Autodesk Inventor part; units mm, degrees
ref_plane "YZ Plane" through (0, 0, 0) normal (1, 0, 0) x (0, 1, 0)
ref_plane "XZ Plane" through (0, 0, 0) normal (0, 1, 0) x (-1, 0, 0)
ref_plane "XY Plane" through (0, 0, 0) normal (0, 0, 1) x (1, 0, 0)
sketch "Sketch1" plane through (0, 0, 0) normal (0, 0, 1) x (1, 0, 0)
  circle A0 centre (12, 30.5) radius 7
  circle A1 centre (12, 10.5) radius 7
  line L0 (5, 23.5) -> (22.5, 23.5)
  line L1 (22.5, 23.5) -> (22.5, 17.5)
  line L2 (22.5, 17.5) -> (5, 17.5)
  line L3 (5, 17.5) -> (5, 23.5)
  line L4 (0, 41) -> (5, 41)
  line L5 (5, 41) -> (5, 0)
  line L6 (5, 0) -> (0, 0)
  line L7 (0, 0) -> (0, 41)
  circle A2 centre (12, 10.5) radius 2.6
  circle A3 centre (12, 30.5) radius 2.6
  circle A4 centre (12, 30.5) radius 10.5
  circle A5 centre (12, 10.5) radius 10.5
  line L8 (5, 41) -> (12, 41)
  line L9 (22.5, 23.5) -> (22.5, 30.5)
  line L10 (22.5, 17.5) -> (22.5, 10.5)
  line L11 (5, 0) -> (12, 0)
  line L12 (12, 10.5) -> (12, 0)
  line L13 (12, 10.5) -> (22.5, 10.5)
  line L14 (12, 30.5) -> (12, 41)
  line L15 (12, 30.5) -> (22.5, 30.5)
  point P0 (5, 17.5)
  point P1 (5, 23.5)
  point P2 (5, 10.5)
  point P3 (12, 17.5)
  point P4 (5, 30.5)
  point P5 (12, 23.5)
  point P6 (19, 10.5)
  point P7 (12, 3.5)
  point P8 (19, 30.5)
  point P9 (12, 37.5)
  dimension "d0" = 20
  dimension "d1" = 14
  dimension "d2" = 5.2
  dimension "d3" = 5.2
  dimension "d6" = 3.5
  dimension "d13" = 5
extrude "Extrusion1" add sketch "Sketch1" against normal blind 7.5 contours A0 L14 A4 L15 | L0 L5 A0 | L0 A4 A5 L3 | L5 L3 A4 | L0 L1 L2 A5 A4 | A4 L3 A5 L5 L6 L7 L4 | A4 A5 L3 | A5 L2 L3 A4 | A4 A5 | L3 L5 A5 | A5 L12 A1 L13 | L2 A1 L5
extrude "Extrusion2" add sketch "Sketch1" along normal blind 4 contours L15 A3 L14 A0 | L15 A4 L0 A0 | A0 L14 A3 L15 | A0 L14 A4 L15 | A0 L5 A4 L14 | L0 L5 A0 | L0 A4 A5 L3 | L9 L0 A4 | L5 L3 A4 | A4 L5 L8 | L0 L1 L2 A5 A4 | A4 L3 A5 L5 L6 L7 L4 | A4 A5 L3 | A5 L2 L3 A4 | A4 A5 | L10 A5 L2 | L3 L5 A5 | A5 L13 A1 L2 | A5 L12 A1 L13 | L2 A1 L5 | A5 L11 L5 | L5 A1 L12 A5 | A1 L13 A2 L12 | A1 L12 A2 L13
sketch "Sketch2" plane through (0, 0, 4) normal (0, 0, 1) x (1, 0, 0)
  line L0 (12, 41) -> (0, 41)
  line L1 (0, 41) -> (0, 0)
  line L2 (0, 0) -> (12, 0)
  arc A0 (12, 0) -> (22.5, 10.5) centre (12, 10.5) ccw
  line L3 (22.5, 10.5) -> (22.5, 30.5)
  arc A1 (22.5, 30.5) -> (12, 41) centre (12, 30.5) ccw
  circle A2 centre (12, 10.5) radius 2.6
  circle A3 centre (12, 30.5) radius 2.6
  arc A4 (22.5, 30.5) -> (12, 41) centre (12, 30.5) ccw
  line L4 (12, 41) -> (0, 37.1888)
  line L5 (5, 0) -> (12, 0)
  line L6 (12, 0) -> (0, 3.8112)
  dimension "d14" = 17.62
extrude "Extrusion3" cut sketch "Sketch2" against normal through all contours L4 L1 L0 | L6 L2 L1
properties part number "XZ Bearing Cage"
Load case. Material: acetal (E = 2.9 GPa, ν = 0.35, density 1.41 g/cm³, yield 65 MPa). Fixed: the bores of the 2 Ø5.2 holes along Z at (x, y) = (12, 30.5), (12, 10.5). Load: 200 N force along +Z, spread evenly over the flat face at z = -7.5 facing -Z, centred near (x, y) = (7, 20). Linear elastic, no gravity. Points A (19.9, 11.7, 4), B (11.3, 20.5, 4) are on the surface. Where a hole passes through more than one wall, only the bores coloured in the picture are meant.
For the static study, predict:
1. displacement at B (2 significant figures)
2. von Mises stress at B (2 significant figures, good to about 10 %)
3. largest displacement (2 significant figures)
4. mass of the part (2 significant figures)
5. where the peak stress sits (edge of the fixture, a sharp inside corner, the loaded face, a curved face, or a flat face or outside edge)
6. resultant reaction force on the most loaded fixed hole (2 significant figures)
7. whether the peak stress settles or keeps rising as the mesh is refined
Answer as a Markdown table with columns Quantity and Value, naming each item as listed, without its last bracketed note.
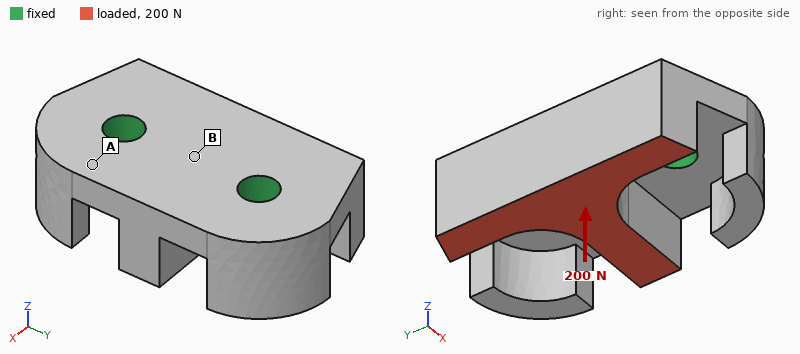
| Quantity | Value |
|---|---|
| displacement at B | 13 µm |
| von Mises stress at B | 2.4 MPa |
| largest displacement | 64 µm |
| mass of the part | 8.6 g |
| where the peak stress sits | edge of the fixture |
| resultant reaction force on the most loaded fixed hole | 100 N |
| whether the peak stress settles or keeps rising as the mesh is refined | keeps rising |
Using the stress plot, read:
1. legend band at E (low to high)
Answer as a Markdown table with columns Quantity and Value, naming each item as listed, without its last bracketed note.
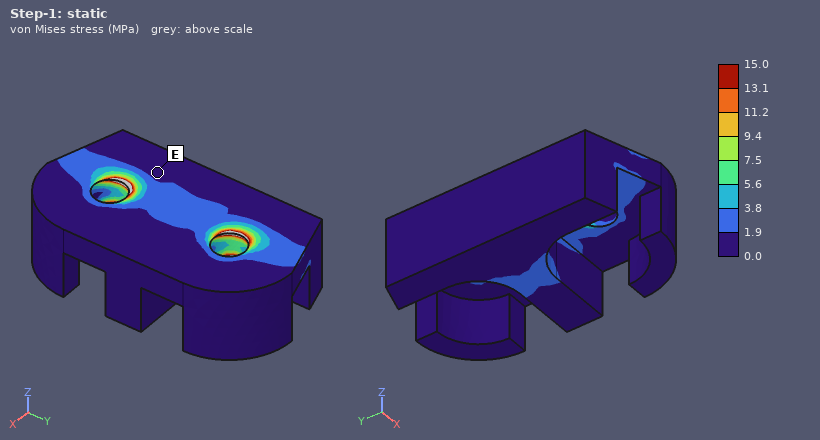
| Quantity | Value |
|---|---|
| legend band at E | 0.0 to 1.9 MPa |
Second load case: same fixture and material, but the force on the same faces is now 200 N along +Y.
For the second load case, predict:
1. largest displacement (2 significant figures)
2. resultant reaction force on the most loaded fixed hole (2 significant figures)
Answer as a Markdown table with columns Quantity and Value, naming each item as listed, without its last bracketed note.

| Quantity | Value |
|---|---|
| largest displacement | 50 µm |
| resultant reaction force on the most loaded fixed hole | 150 N |
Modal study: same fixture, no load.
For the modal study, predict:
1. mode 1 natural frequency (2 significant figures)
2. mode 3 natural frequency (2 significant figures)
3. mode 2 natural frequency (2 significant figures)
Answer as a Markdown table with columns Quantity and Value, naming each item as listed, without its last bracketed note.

| Quantity | Value |
|---|---|
| mode 1 natural frequency | 3900 Hz |
| mode 3 natural frequency | 5300 Hz |
| mode 2 natural frequency | 5200 Hz |
